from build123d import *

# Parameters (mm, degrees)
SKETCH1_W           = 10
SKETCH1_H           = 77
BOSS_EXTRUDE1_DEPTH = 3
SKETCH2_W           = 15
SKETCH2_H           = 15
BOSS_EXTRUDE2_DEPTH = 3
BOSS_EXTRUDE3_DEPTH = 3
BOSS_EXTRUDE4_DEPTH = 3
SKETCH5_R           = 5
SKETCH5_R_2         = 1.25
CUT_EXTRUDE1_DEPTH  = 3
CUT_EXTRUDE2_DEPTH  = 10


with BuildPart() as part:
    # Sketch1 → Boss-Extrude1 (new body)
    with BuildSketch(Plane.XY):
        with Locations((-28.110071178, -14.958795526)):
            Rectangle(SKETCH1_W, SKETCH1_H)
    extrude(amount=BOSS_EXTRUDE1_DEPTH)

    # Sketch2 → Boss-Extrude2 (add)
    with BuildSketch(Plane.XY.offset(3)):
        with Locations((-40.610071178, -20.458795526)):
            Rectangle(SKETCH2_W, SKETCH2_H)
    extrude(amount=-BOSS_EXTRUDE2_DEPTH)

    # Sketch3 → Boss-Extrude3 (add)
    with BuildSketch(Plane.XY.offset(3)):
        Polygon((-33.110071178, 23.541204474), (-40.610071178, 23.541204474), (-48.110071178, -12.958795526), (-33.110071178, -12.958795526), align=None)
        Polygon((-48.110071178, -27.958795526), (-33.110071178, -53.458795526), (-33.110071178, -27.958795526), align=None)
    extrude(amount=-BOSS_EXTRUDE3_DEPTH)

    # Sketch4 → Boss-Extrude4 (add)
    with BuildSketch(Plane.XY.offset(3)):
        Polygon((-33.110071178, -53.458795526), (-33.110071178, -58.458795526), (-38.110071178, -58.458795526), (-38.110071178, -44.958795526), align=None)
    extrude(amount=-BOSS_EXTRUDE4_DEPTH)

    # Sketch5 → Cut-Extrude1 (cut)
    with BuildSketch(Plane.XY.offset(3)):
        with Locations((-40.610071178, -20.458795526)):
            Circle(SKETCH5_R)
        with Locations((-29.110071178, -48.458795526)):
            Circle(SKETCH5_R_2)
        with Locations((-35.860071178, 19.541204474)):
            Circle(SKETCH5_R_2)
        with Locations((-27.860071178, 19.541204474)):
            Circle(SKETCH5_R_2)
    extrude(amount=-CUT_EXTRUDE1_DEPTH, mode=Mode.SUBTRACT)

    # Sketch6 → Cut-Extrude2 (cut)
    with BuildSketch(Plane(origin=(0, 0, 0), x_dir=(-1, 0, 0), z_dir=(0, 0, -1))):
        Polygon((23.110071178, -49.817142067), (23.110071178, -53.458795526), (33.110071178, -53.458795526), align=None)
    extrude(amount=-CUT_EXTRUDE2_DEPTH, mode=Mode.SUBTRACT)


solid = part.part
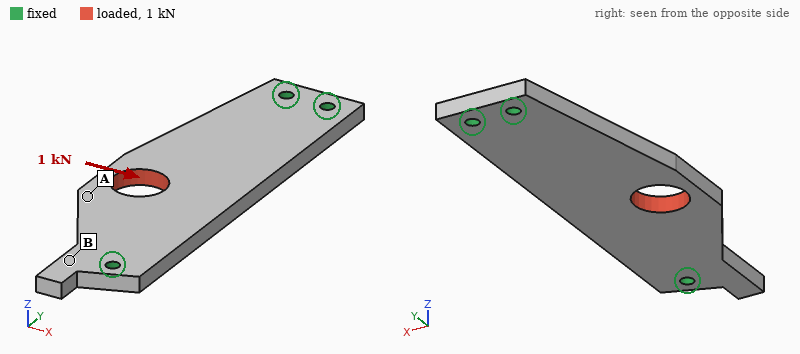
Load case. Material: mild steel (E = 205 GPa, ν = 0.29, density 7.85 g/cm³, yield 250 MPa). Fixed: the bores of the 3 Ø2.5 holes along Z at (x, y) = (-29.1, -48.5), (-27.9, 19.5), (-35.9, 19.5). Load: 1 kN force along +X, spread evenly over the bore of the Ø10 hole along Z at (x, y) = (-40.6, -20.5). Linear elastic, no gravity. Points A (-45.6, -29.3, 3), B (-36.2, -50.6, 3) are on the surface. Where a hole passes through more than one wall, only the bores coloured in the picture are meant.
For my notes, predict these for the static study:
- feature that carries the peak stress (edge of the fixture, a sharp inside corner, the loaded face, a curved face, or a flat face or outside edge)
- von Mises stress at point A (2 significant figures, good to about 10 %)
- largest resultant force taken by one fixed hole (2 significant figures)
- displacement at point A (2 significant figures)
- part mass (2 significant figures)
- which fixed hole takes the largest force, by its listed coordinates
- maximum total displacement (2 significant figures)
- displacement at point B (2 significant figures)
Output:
edge of the fixture
35 MPa
770 N
8.3 µm
36 g
(-27.9, 19.5)
9.8 µm
2.0 µm
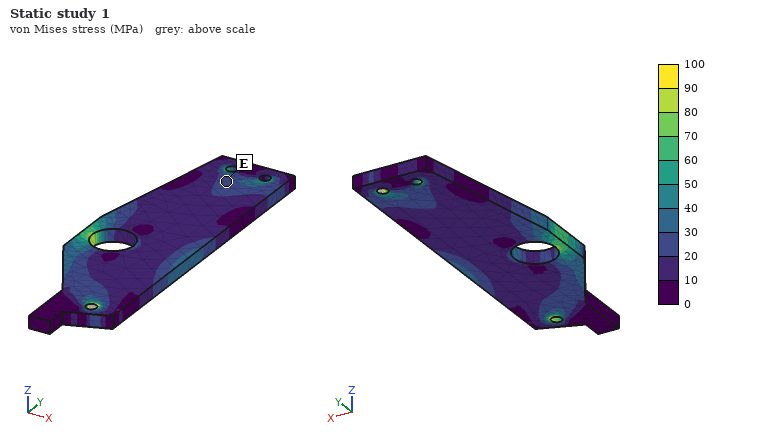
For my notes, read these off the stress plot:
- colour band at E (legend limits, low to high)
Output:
20 to 30 MPa
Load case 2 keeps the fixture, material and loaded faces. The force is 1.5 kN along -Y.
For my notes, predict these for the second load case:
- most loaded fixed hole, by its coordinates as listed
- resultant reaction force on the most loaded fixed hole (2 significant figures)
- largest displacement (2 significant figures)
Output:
(-29.1, -48.5)
730 N
4.4 µm
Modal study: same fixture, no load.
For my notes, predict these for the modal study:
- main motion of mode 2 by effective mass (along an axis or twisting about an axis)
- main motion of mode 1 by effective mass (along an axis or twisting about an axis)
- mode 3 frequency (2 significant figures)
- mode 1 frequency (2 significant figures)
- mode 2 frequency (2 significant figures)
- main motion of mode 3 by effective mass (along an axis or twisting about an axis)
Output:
twisting about Y
along Z
8100 Hz
2900 Hz
5500 Hz
twisting about X
